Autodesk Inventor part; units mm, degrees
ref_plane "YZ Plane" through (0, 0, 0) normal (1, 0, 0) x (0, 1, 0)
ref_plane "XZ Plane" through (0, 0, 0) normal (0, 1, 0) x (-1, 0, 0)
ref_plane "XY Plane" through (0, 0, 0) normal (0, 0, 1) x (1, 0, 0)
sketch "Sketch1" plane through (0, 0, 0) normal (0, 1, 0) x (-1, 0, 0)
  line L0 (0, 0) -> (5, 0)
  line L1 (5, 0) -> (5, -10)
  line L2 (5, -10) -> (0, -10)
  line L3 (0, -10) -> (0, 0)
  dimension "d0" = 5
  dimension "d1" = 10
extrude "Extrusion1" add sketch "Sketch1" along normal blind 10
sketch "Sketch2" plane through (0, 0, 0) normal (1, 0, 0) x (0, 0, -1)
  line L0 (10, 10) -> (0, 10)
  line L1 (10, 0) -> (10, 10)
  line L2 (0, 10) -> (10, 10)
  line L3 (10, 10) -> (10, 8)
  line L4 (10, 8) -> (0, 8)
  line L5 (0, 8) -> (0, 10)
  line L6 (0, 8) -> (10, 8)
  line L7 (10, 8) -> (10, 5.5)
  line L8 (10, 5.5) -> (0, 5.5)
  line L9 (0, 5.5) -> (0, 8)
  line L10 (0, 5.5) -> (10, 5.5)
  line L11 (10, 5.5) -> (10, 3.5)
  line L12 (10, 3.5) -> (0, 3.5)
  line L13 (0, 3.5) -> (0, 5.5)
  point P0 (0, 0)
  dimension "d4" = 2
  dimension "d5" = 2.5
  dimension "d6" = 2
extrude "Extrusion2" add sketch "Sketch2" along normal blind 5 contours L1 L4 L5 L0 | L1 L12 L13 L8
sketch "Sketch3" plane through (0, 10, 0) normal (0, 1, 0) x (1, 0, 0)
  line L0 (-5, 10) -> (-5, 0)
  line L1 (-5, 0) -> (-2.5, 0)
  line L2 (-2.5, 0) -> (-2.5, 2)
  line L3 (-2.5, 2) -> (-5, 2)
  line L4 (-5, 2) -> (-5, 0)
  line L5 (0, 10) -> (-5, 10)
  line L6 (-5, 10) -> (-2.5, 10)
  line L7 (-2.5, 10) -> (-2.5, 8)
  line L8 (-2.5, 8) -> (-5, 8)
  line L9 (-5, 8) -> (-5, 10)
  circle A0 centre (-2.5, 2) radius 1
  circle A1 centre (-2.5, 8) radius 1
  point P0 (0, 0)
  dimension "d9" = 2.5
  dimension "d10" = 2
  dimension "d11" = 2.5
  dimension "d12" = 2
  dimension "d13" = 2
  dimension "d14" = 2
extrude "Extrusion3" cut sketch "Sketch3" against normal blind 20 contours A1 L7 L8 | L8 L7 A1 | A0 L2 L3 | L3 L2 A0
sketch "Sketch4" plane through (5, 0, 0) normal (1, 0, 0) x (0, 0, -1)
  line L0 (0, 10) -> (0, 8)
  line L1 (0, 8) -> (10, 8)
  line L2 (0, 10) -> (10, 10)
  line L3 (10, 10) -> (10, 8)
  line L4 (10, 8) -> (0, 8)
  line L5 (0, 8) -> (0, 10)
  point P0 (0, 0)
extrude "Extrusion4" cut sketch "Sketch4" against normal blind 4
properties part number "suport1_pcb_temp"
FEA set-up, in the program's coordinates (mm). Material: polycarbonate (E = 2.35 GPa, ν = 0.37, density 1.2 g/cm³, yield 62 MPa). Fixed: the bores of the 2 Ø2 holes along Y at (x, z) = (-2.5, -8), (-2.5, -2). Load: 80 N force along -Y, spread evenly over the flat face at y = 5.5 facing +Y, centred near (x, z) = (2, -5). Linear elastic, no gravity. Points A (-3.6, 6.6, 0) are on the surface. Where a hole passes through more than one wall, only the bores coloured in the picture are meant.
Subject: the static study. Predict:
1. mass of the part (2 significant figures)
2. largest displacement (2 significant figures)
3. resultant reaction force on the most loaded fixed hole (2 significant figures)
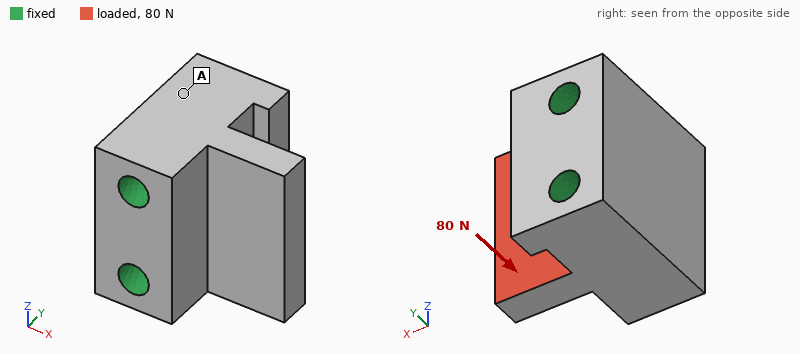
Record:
0.67 g
0.14 mm
40 N
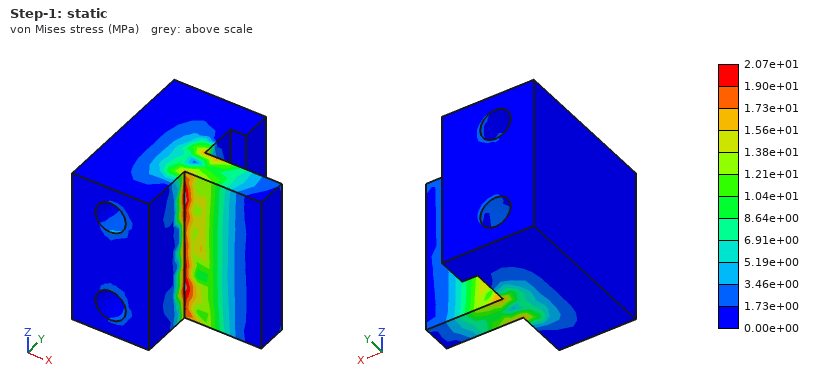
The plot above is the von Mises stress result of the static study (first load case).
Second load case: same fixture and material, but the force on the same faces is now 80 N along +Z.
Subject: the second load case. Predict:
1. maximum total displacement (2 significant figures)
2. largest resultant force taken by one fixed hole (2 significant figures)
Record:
51 µm
63 N
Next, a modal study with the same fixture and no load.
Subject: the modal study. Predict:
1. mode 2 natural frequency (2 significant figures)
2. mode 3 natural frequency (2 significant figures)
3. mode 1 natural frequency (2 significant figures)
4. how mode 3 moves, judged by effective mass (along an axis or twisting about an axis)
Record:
20 kHz
27 kHz
14 kHz
along Z
